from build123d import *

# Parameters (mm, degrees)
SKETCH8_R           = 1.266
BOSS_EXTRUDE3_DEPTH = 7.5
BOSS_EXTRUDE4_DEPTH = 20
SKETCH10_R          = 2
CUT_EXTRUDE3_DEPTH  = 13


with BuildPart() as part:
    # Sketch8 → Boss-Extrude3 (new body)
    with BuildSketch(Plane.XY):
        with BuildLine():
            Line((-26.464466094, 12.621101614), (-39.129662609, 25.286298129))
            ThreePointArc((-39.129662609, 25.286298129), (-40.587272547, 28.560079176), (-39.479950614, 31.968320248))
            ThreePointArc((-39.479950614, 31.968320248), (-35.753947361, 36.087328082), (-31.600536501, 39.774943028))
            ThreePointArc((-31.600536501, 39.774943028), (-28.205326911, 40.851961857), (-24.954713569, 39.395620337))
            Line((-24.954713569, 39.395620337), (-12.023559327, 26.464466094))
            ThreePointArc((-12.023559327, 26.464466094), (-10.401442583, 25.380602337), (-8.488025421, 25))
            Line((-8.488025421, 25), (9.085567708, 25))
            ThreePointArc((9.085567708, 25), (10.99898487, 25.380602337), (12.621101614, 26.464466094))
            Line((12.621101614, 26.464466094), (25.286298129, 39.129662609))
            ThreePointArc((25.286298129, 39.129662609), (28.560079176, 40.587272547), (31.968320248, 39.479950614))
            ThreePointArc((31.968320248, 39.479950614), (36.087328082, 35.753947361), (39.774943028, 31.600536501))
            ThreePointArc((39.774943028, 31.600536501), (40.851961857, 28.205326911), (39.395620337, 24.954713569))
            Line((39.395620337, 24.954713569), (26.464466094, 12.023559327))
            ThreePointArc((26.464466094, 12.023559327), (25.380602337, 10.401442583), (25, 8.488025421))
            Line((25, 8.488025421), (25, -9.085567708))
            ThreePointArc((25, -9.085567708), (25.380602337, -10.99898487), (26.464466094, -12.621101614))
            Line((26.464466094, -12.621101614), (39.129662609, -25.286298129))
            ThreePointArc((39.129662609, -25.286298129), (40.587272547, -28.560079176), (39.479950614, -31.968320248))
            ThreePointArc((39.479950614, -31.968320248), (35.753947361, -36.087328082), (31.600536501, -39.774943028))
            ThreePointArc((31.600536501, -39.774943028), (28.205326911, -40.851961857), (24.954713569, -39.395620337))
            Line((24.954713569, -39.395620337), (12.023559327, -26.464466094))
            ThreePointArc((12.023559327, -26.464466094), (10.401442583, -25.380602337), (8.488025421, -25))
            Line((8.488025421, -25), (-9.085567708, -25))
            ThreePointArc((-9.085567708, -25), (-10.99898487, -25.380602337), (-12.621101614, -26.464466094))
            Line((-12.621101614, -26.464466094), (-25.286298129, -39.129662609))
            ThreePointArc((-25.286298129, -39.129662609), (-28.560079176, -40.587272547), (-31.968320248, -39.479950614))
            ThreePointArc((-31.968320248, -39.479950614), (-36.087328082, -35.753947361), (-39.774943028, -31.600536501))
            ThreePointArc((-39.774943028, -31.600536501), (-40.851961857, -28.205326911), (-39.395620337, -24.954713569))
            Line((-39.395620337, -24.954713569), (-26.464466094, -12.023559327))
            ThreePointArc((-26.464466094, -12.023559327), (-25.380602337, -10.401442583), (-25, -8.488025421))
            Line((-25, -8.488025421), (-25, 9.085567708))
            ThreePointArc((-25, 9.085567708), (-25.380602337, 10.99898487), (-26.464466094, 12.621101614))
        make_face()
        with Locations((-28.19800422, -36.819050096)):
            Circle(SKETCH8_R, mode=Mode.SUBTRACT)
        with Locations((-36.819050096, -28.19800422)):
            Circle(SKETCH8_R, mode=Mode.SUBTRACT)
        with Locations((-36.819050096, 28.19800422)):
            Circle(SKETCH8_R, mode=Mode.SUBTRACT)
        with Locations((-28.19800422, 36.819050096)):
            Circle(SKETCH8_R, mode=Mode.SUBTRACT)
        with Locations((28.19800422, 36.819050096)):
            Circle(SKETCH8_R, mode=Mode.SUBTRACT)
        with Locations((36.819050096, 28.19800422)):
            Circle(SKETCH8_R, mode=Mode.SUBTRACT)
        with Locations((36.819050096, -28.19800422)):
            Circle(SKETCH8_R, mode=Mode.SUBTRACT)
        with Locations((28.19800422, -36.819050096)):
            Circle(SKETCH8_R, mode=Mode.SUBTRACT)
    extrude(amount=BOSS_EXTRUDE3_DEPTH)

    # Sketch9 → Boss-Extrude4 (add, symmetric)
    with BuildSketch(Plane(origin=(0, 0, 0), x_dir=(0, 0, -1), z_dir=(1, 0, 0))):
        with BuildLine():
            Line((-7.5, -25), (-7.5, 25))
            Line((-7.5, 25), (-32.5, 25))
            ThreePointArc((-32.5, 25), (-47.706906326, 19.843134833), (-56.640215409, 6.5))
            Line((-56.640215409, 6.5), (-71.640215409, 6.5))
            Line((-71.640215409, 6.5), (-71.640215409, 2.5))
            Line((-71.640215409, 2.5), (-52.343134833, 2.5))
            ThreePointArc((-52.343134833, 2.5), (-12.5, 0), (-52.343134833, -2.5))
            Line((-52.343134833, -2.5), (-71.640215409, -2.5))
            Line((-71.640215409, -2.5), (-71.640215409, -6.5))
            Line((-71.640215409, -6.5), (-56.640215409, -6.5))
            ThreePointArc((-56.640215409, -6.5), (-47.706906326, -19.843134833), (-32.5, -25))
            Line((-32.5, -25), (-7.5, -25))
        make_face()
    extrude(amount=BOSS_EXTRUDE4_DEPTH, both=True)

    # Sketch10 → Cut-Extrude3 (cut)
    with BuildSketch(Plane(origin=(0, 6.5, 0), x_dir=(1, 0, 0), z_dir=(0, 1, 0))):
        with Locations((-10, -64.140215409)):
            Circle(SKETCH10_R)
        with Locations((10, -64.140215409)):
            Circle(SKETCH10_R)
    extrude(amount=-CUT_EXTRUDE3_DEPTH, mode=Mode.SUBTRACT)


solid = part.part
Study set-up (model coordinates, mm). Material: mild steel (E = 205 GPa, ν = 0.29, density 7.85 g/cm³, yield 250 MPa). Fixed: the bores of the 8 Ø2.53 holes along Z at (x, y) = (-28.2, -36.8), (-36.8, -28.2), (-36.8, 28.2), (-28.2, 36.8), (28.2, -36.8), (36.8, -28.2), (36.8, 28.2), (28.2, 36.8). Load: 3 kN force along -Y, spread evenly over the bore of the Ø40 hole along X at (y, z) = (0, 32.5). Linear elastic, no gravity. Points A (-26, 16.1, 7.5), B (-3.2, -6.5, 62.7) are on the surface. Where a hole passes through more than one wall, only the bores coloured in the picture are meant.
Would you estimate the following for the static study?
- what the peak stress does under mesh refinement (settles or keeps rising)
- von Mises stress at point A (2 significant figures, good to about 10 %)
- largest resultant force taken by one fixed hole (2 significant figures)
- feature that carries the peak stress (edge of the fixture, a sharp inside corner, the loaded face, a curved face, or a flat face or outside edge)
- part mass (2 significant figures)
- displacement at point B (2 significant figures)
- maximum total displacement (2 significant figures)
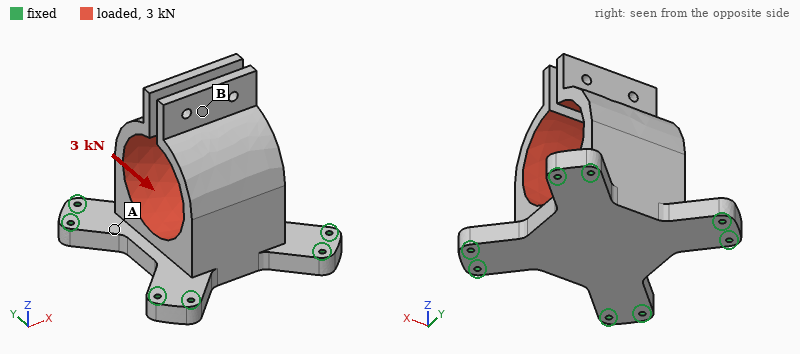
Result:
keeps rising
20 MPa
850 N
edge of the fixture
570 g
0.090 mm
0.11 mm
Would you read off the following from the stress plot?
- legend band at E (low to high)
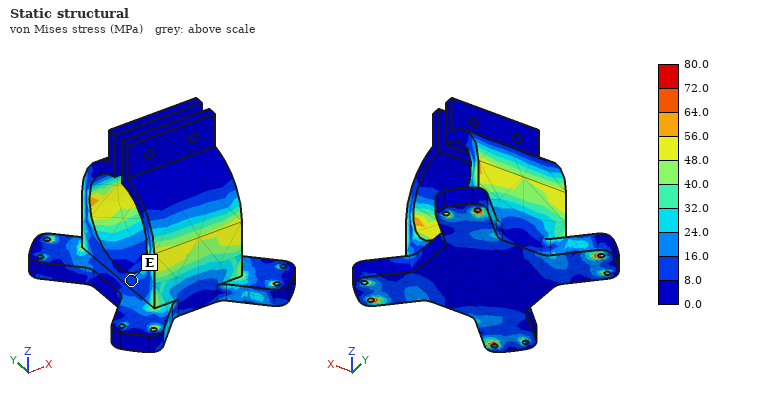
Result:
8.0 to 16.0 MPa
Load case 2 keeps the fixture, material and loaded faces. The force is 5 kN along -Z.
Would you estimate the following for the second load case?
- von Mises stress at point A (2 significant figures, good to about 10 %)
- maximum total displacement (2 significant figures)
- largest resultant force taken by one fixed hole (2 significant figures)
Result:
24 MPa
0.13 mm
790 N
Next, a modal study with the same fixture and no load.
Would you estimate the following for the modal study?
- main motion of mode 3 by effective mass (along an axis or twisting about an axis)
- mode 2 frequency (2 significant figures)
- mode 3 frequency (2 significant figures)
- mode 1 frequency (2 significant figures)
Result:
along X
1500 Hz
3200 Hz
1500 Hz
